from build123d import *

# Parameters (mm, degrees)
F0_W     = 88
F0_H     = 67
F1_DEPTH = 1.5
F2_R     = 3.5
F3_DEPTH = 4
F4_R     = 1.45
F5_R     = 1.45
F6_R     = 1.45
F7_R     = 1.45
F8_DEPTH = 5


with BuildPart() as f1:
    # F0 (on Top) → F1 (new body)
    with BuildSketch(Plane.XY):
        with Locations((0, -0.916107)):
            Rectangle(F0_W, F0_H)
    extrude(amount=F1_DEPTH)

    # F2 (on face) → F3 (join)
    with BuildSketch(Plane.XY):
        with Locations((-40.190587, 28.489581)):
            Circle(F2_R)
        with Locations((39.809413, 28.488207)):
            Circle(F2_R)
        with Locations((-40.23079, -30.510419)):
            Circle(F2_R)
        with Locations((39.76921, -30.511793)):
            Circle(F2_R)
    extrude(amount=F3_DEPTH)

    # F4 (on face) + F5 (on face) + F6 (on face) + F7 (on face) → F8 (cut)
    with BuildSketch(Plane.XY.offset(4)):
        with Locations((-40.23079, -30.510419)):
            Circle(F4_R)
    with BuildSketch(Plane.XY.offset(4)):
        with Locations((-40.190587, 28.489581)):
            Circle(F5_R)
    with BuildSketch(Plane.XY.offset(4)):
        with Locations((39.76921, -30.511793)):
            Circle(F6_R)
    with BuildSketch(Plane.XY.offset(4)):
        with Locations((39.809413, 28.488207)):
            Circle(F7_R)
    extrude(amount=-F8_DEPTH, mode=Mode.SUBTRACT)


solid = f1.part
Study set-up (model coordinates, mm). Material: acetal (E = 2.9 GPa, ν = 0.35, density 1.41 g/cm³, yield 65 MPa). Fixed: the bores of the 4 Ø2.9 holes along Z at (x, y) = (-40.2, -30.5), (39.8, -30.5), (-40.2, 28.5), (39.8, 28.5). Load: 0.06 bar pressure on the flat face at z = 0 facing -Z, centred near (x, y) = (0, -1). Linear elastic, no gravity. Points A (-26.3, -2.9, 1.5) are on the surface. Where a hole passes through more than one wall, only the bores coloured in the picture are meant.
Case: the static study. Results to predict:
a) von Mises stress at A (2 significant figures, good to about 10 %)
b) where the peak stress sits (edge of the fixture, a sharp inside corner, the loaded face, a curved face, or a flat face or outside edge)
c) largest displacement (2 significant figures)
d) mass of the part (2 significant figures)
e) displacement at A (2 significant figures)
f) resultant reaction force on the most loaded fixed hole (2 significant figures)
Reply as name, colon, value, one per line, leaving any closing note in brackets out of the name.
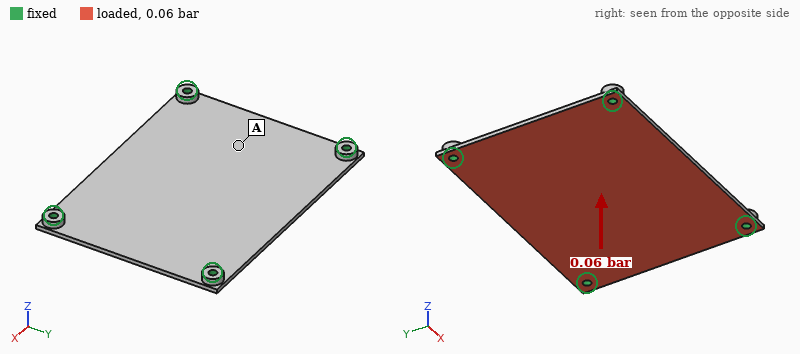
von Mises stress at A: 2.8 MPa
where the peak stress sits: the loaded face
largest displacement: 1.1 mm
mass of the part: 13 g
displacement at A: 0.65 mm
resultant reaction force on the most loaded fixed hole: 10 N
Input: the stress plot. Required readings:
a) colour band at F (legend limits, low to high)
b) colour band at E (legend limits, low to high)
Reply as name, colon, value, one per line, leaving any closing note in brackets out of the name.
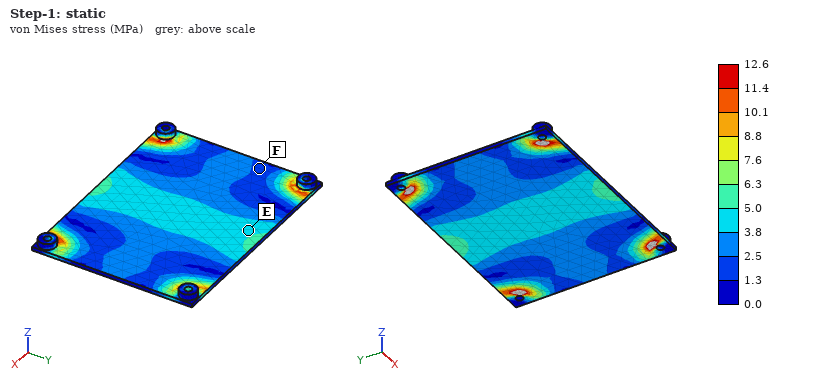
colour band at F: 1.3 to 2.5 MPa
colour band at E: 3.8 to 5.0 MPa
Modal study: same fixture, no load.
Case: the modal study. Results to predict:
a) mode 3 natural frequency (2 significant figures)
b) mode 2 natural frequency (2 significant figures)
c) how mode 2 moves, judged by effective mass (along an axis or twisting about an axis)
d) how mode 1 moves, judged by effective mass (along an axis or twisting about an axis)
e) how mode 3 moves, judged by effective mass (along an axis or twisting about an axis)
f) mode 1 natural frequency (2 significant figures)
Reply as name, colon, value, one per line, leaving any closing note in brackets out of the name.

mode 3 natural frequency: 670 Hz
mode 2 natural frequency: 470 Hz
how mode 2 moves, judged by effective mass: twisting about X
how mode 1 moves, judged by effective mass: along Z
how mode 3 moves, judged by effective mass: twisting about Y
mode 1 natural frequency: 300 Hz
